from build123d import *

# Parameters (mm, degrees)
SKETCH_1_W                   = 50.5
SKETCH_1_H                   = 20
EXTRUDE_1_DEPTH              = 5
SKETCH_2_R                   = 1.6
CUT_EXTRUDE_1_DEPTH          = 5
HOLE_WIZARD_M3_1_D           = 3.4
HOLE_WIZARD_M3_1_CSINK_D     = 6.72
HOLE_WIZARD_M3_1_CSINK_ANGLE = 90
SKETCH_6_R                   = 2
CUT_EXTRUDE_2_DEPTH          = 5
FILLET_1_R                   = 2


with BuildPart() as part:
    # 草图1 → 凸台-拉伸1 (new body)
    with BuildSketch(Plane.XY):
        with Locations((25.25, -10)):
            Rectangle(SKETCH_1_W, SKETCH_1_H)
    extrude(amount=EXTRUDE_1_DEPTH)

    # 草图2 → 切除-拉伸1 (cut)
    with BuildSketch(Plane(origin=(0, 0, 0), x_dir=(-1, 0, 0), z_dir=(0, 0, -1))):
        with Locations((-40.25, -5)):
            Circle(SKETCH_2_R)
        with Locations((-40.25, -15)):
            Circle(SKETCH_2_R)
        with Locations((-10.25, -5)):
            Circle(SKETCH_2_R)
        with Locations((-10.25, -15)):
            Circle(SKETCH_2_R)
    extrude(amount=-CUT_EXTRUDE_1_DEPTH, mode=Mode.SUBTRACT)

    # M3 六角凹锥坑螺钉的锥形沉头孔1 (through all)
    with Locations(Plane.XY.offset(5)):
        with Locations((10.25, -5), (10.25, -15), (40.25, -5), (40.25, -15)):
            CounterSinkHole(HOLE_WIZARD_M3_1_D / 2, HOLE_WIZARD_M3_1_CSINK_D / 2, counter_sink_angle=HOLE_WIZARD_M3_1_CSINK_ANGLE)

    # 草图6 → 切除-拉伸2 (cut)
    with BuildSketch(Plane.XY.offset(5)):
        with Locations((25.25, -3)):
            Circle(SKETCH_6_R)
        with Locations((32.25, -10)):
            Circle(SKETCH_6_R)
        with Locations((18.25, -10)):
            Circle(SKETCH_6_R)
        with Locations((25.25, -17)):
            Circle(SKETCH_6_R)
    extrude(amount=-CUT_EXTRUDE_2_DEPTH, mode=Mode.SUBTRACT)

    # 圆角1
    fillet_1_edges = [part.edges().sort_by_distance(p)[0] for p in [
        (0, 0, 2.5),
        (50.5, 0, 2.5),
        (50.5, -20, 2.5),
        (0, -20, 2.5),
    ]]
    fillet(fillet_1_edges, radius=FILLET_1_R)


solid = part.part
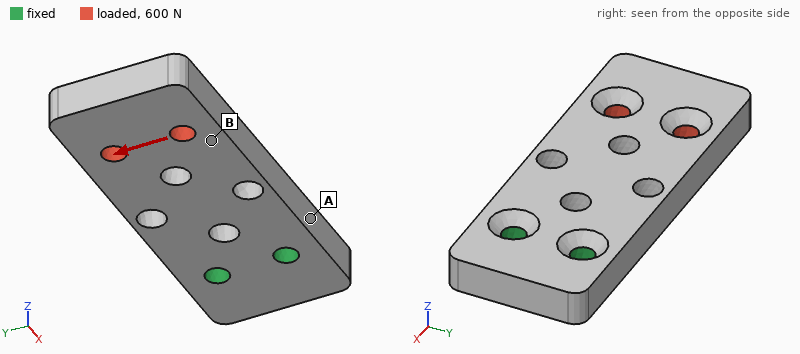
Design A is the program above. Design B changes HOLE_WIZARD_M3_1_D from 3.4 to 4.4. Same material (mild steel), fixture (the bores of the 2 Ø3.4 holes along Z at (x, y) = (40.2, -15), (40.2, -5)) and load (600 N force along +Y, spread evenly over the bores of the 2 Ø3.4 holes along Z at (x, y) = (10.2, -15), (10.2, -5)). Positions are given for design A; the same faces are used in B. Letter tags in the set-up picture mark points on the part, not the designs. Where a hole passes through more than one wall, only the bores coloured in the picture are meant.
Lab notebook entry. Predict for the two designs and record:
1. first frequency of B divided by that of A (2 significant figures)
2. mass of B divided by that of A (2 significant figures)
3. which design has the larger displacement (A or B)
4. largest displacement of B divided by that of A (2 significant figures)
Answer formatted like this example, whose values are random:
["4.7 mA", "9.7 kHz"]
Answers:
["1.1", "0.98", "A", "0.90"]
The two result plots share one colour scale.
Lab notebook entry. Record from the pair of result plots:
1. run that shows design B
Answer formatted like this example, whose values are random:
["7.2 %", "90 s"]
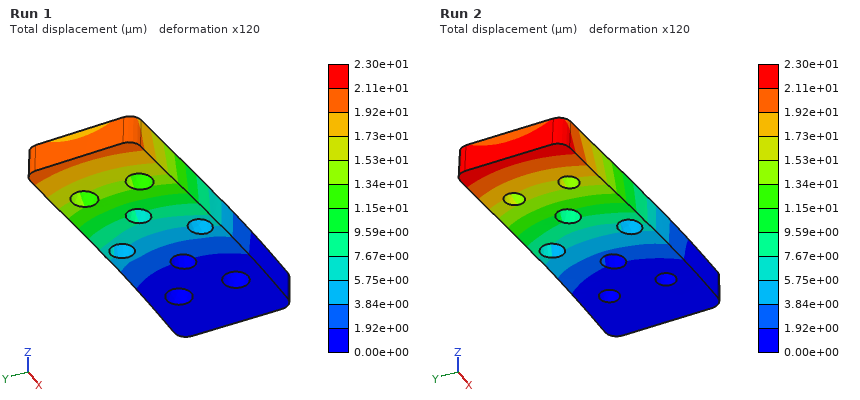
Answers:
["Run 1"]
